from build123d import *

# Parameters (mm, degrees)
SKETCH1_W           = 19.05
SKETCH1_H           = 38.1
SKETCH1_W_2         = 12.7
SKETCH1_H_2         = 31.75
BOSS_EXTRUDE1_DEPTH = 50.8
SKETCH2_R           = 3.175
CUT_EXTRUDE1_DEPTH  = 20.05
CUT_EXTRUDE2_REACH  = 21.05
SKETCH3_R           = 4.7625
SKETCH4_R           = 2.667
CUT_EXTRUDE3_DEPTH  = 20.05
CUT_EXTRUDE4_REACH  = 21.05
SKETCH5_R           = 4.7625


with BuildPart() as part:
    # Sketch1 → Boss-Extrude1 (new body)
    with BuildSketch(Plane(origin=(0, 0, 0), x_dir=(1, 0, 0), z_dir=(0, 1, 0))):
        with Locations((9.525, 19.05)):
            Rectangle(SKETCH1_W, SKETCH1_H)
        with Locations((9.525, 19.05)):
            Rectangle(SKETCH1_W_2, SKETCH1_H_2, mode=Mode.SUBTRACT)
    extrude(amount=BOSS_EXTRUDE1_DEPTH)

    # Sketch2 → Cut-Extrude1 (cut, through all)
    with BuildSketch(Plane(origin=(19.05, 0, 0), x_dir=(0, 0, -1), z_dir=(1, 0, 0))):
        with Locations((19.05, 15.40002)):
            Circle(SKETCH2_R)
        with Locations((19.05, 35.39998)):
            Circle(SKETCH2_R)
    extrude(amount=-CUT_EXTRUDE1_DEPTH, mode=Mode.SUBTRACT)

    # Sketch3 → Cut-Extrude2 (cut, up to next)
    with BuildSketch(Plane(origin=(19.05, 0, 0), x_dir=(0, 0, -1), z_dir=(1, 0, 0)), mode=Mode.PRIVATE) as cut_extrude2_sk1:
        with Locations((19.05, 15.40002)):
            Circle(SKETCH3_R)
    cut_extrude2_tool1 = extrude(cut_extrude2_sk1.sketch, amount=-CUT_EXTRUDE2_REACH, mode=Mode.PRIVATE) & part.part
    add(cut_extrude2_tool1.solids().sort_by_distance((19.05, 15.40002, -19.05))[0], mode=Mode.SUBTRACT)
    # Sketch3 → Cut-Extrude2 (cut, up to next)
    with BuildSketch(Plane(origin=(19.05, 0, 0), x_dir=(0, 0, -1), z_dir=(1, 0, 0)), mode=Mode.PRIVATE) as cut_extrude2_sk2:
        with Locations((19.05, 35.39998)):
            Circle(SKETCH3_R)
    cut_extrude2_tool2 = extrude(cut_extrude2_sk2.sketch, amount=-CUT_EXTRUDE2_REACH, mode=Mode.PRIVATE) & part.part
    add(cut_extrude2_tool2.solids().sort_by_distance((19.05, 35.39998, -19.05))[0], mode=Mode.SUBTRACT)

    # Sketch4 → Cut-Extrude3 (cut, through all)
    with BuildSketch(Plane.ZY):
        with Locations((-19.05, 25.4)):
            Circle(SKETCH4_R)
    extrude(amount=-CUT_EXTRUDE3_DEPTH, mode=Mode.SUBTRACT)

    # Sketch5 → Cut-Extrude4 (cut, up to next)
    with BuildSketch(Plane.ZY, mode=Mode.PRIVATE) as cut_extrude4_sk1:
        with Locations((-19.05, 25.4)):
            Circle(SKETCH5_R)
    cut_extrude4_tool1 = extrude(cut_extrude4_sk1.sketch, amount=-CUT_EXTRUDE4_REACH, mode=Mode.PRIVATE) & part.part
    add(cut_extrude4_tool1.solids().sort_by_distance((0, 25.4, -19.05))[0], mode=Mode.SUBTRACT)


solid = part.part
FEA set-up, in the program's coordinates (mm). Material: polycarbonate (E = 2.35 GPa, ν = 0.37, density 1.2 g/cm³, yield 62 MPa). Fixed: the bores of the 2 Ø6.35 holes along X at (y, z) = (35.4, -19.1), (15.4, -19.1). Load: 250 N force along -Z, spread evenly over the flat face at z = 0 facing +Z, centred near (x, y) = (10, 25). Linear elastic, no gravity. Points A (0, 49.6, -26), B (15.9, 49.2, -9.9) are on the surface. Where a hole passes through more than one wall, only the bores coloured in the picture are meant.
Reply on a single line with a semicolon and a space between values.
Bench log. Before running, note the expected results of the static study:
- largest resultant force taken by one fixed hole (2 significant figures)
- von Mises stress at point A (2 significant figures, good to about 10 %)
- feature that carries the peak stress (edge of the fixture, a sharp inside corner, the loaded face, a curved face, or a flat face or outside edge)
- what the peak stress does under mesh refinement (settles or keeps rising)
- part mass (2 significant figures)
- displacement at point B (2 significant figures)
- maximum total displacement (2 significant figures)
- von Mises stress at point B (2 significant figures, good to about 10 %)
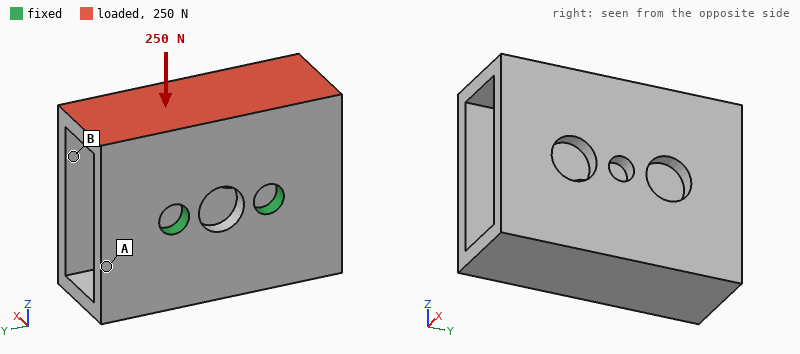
130 N; 5.7 MPa; edge of the fixture; keeps rising; 19 g; 0.57 mm; 0.74 mm; 2.2 MPa
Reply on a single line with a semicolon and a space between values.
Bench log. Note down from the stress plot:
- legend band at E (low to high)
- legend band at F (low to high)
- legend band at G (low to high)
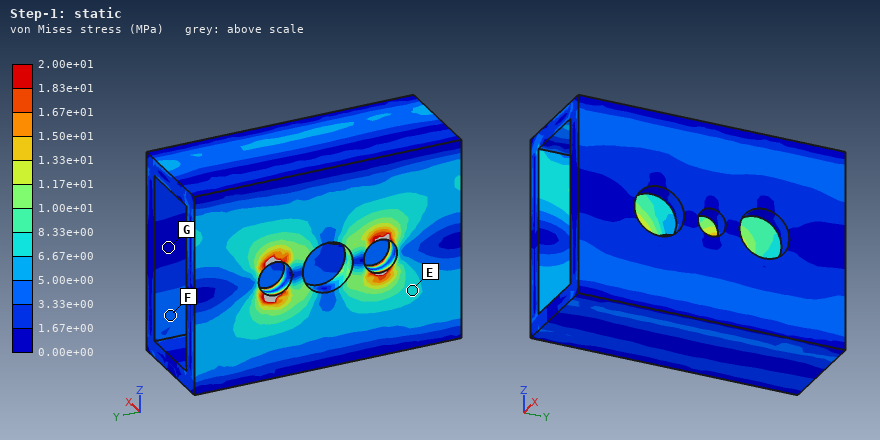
6.67e+00 to 8.33e+00 MPa; 3.33e+00 to 5.00e+00 MPa; 0.00e+00 to 1.67e+00 MPa
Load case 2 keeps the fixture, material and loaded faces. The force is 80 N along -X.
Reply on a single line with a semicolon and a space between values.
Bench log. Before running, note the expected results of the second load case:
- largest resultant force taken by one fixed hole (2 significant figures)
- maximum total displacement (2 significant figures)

40 N; 0.42 mm
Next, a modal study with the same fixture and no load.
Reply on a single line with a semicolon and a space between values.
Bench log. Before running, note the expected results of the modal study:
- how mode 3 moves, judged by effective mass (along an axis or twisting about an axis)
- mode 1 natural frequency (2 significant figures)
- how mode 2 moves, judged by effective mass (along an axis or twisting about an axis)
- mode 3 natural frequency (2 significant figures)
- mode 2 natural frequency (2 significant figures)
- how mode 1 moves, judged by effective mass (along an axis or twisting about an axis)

along X; 670 Hz; along Y; 1300 Hz; 1000 Hz; along Z
